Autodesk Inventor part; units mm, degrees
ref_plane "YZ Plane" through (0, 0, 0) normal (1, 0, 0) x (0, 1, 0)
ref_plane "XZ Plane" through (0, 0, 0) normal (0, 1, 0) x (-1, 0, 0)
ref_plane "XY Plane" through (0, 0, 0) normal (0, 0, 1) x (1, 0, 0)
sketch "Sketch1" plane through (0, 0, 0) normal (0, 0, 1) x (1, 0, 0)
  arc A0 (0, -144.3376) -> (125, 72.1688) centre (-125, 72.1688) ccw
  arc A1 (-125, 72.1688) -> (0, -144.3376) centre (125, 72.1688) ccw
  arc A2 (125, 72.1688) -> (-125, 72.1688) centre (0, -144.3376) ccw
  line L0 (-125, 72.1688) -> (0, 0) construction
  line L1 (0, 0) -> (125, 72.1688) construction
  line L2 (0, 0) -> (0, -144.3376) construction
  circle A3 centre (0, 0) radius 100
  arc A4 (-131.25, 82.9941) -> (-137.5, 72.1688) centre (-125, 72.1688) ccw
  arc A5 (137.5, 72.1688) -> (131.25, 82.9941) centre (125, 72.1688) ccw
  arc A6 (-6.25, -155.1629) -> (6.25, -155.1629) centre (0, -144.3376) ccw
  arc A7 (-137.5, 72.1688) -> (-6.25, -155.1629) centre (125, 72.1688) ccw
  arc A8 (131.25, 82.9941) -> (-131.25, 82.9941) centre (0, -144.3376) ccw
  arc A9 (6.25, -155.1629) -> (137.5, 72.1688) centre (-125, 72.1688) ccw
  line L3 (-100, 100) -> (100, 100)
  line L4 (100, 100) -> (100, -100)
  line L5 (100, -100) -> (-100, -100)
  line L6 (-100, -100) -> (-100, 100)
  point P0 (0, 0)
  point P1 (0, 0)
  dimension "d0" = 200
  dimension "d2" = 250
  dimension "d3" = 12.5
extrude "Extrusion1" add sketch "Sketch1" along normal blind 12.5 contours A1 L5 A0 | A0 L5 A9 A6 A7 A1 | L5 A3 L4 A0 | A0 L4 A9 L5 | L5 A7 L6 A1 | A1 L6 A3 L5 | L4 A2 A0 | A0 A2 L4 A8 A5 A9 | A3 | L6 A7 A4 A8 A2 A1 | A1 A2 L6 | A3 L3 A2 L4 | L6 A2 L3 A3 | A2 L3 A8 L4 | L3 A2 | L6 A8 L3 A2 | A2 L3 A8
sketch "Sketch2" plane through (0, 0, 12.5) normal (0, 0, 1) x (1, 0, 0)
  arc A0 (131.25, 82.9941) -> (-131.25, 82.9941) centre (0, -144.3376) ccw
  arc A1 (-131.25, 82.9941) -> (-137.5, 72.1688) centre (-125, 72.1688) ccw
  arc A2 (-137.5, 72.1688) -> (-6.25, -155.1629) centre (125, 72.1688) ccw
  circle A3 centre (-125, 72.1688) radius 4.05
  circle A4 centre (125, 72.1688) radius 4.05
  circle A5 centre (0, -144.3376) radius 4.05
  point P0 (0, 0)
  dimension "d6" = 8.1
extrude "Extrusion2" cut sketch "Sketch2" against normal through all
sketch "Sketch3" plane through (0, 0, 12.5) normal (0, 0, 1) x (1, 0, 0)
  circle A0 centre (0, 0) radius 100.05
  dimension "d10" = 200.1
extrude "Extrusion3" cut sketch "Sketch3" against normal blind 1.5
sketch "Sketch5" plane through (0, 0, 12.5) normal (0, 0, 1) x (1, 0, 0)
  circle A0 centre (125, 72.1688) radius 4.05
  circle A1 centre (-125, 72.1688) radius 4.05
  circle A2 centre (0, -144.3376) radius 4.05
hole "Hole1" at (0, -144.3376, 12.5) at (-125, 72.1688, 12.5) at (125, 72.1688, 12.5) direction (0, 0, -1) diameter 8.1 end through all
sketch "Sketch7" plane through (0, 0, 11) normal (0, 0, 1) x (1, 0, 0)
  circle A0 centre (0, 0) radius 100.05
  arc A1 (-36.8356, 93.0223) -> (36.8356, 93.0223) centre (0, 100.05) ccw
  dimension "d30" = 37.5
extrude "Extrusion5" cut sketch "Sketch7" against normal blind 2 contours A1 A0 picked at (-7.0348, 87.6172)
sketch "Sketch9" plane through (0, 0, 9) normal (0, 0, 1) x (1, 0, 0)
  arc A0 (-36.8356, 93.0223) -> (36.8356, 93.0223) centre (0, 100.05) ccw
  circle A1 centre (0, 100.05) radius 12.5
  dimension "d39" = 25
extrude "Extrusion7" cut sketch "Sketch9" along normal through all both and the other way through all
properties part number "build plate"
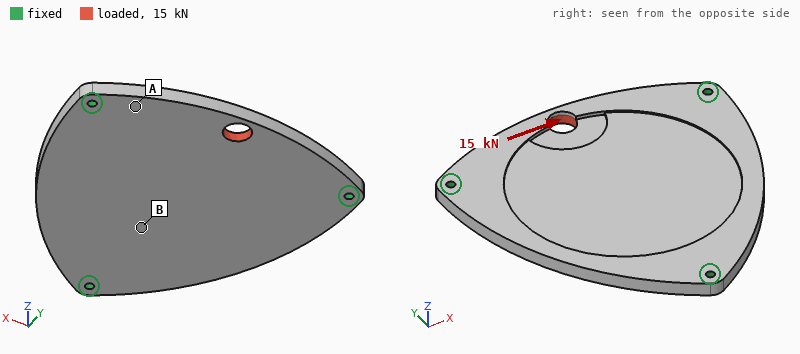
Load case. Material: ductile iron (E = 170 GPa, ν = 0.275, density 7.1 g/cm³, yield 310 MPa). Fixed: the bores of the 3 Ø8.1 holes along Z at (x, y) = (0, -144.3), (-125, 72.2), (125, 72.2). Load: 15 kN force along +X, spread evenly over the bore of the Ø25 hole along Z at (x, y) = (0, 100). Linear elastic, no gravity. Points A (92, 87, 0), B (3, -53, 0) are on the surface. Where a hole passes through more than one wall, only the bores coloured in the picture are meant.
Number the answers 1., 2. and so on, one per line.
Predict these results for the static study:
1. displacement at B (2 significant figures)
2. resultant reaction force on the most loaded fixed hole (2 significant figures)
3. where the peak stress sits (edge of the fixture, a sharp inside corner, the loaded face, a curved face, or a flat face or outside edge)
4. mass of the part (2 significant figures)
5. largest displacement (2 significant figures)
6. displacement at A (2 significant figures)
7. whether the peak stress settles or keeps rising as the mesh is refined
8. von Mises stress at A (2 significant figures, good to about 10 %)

1. 2.5 µm
2. 7.5 kN
3. edge of the fixture
4. 4.4 kg
5. 15 µm
6. 3.8 µm
7. keeps rising
8. 14 MPa
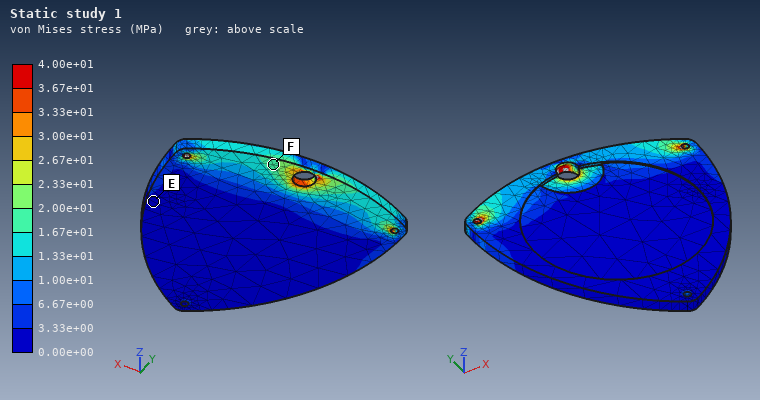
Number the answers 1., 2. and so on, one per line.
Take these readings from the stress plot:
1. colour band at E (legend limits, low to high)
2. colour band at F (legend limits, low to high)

1. 0.00e+00 to 3.33e+00 MPa
2. 1.67e+01 to 2.00e+01 MPa
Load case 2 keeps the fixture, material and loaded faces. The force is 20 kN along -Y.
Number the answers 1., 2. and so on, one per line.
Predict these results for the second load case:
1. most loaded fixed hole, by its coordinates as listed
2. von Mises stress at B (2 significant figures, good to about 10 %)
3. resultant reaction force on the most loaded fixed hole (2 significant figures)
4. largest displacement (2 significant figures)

1. (0, -144.3)
2. 11 MPa
3. 8.1 kN
4. 40 µm
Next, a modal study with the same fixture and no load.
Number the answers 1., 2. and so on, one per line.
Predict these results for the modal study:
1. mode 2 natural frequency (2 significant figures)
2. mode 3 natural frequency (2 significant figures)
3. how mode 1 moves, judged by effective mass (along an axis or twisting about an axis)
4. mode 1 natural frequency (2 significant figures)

1. 940 Hz
2. 950 Hz
3. along Z
4. 710 Hz
